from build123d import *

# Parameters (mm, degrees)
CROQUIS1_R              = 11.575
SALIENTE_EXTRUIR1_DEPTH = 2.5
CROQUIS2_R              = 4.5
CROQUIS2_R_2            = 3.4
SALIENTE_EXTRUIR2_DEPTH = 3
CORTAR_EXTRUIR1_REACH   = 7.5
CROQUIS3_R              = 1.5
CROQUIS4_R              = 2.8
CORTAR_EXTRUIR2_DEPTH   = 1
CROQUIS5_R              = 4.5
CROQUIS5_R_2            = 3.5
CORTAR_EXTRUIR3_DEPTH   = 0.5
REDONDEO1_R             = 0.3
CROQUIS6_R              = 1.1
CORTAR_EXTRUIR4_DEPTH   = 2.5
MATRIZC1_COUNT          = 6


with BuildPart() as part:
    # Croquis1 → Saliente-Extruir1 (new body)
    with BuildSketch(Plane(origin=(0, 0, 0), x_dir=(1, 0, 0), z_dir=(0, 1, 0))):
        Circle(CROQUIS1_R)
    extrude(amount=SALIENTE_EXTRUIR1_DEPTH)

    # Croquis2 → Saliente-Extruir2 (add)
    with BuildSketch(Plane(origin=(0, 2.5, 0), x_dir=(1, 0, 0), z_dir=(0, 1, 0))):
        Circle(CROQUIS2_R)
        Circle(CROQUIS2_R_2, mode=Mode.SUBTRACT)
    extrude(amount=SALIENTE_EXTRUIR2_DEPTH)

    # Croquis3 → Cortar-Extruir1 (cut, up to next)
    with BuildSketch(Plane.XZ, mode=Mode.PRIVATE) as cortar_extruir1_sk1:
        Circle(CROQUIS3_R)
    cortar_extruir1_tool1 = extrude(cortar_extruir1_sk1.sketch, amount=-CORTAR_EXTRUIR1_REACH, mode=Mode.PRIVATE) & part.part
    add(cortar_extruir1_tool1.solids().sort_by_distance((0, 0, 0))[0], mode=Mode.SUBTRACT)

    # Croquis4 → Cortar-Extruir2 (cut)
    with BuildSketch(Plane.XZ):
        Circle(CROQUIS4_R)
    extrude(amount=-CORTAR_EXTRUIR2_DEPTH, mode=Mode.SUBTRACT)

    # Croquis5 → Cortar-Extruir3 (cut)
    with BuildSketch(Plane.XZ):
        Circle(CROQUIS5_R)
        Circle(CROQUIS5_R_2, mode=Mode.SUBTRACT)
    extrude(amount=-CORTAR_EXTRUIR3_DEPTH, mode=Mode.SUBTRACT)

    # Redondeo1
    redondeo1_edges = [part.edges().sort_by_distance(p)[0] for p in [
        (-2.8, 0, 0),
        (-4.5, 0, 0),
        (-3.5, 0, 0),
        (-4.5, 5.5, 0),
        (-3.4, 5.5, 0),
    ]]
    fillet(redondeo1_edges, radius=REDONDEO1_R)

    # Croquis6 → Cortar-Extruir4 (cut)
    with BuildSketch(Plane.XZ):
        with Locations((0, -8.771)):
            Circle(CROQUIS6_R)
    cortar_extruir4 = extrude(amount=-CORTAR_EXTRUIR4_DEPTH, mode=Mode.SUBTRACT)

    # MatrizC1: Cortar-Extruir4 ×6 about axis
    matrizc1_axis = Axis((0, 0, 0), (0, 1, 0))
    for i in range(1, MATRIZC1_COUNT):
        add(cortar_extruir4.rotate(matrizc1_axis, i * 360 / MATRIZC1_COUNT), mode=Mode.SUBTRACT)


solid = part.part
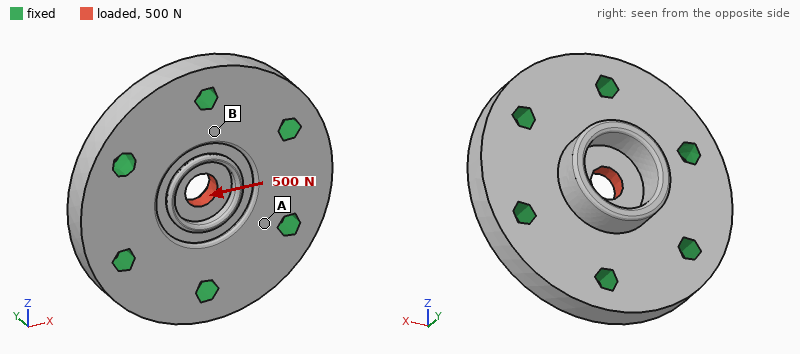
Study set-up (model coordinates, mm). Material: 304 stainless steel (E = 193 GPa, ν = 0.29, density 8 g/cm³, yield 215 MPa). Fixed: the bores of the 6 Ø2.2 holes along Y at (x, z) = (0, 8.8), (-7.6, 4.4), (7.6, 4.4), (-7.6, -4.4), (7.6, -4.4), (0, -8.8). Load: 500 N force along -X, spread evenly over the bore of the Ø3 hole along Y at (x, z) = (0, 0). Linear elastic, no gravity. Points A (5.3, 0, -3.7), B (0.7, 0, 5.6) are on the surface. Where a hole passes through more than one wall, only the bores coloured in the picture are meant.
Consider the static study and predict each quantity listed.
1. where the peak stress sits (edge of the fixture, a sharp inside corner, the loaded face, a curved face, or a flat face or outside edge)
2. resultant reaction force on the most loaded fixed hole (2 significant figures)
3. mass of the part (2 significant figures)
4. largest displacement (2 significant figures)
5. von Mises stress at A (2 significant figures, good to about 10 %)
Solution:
a sharp inside corner
120 N
8.2 g
0.69 µm
9.3 MPa
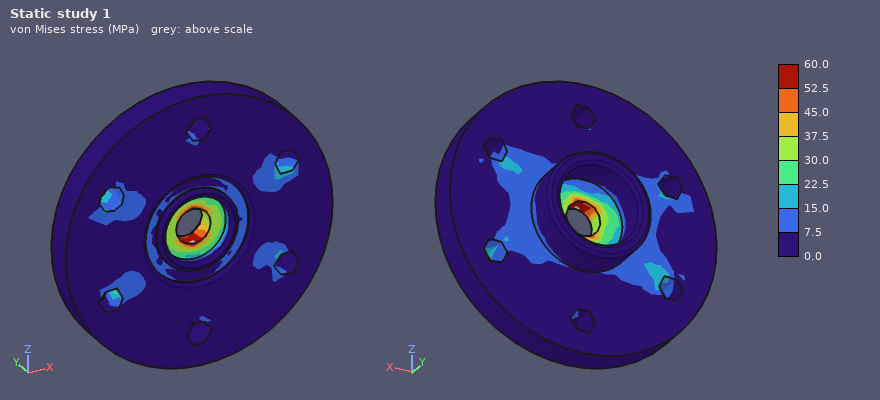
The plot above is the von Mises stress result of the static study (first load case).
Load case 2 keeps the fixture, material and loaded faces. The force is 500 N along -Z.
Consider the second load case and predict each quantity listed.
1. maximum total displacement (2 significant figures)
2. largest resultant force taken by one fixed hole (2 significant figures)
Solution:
0.68 µm
130 N
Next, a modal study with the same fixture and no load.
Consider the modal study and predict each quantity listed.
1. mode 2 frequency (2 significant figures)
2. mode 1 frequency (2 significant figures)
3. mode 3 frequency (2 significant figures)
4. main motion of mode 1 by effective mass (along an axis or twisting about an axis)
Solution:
92 kHz
66 kHz
92 kHz
along Y
